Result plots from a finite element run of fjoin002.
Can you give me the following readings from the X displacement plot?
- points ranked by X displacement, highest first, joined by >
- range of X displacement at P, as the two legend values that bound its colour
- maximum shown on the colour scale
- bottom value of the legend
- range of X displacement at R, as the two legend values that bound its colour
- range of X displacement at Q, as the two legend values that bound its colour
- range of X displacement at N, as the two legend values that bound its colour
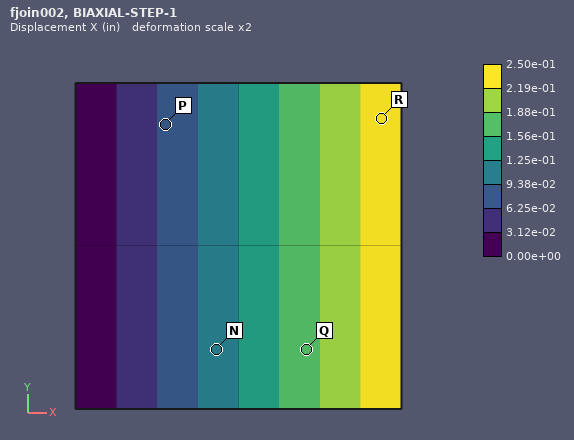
R > Q > N > P
6.25e-02 to 9.38e-02 in
2.50e-01 in
0.00e+00 in
2.19e-01 to 2.50e-01 in
1.56e-01 to 1.88e-01 in
9.38e-02 to 1.25e-01 in
